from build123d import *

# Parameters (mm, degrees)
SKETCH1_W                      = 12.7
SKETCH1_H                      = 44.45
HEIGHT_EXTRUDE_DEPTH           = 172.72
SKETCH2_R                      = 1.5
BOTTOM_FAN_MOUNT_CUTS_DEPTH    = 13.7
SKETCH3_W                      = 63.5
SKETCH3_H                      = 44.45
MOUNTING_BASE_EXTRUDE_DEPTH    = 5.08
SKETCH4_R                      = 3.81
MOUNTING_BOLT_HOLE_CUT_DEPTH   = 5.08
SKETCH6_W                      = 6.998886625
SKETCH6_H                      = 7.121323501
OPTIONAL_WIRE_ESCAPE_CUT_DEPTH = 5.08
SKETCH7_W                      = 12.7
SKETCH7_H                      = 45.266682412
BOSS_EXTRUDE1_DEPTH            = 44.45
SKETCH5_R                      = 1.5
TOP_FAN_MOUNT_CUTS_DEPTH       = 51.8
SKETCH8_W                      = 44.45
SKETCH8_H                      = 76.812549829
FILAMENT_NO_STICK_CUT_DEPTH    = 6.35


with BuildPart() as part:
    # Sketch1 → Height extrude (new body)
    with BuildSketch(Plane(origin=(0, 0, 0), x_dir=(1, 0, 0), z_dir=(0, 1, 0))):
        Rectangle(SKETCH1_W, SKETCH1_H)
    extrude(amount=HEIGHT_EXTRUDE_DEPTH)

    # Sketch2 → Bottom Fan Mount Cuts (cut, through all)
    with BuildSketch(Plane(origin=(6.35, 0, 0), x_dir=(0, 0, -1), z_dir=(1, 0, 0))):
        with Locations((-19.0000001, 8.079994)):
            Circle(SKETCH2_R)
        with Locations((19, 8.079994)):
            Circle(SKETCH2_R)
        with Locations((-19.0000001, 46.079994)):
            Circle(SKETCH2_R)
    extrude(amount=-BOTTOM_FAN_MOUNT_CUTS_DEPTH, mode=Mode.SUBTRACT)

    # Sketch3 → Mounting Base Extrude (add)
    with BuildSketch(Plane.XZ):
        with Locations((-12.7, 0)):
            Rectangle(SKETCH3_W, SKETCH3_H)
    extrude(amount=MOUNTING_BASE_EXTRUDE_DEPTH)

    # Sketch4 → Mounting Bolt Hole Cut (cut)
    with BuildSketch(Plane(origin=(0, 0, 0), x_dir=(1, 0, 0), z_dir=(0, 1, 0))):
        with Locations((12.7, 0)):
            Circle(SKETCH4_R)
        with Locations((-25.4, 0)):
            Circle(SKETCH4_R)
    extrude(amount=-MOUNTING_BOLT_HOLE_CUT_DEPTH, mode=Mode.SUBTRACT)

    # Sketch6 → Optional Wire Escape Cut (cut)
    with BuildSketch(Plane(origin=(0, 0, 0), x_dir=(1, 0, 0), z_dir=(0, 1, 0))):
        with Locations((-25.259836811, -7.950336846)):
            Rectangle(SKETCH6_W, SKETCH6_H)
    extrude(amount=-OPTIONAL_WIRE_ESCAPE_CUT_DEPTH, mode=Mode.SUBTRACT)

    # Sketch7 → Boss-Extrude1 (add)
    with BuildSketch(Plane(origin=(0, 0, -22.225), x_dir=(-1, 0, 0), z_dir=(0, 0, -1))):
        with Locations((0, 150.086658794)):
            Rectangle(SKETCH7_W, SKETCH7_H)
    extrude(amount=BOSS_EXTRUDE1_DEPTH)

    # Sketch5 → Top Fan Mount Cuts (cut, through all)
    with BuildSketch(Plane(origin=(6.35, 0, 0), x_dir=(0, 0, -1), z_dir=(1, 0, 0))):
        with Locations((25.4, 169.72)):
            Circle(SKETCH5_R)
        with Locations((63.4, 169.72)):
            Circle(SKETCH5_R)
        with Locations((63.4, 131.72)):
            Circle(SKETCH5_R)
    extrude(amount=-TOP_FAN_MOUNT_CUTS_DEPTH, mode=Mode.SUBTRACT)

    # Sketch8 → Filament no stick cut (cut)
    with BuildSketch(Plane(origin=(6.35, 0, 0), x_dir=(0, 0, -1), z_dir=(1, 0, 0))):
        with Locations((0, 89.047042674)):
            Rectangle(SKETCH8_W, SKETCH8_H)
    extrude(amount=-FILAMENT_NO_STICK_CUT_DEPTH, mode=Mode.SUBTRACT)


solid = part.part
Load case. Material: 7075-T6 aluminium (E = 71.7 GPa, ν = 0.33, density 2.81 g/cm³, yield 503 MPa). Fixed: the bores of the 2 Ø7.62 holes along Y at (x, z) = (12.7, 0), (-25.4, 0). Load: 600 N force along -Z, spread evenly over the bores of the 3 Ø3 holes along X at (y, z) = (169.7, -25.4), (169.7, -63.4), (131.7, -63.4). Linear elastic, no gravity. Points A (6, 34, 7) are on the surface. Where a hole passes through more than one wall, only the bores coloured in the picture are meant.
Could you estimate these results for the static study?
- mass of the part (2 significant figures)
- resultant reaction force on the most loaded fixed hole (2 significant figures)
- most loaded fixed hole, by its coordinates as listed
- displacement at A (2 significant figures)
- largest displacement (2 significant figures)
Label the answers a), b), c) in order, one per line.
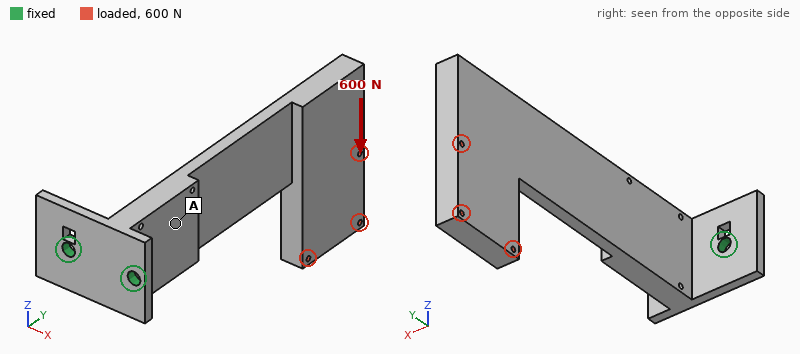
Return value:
a) 320 g
b) 570 N
c) (12.7, 0)
d) 0.32 mm
e) 1.8 mm
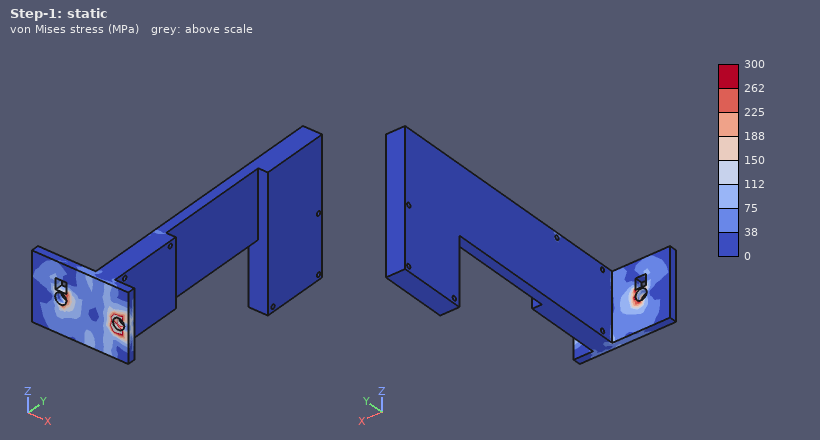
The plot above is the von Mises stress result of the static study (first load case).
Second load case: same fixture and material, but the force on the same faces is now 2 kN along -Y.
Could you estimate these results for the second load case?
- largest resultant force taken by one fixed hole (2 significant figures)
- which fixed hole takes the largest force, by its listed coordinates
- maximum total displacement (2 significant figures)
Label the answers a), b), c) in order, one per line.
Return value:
a) 1.4 kN
b) (12.7, 0)
c) 2.2 mm
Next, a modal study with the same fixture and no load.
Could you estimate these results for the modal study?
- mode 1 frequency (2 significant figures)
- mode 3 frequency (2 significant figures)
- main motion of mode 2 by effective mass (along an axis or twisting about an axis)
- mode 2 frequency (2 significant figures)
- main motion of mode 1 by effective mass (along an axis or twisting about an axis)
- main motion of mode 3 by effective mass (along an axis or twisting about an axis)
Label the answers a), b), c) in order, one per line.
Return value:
a) 140 Hz
b) 560 Hz
c) along Z
d) 250 Hz
e) along X
f) twisting about Y
